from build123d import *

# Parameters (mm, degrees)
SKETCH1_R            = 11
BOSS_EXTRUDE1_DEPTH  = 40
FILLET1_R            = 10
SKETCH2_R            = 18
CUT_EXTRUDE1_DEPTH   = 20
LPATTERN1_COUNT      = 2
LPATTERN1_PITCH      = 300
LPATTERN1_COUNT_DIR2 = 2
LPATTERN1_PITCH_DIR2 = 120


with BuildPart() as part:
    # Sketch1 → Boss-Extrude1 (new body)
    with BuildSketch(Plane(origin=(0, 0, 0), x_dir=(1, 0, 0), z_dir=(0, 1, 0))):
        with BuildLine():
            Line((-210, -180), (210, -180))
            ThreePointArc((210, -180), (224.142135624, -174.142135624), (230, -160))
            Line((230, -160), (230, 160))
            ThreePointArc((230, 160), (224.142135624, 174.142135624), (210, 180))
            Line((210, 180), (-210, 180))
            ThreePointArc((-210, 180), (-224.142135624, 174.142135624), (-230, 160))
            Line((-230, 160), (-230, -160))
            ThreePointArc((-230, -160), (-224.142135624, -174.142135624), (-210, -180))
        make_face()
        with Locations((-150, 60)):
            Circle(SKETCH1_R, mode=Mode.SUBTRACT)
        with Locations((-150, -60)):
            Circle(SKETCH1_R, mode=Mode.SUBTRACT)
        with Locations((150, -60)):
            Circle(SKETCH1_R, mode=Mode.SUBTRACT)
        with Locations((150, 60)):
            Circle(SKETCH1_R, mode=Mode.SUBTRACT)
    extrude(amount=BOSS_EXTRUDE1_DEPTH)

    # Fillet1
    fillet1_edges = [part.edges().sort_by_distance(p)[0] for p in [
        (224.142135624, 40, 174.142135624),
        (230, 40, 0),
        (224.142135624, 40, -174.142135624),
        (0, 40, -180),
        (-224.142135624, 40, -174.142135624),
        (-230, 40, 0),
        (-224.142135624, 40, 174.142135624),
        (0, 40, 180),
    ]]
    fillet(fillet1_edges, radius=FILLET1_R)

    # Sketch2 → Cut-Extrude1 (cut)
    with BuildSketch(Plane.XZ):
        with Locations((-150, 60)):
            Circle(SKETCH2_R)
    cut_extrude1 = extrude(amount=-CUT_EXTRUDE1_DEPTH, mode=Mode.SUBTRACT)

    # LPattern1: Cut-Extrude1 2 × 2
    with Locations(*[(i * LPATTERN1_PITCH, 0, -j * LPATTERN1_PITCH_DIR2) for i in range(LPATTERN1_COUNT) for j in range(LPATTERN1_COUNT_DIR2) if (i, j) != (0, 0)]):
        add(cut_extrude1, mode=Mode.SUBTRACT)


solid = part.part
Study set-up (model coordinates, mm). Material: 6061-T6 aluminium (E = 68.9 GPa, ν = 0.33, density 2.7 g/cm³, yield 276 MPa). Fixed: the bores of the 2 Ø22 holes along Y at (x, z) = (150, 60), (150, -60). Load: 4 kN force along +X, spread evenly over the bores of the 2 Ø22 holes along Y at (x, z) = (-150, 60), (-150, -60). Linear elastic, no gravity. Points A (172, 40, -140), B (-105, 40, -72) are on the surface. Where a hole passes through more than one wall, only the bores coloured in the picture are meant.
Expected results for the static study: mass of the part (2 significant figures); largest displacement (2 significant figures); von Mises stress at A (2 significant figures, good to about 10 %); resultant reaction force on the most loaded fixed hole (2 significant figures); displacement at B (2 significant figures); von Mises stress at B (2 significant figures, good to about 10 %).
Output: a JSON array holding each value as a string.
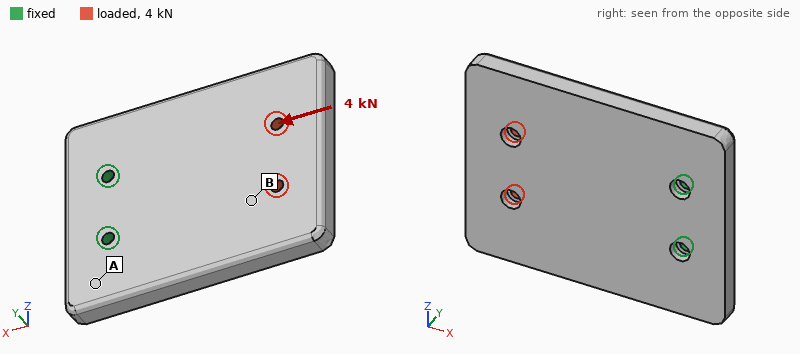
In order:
["17 kg", "19 µm", "0.20 MPa", "2.0 kN", "9.2 µm", "0.96 MPa"]
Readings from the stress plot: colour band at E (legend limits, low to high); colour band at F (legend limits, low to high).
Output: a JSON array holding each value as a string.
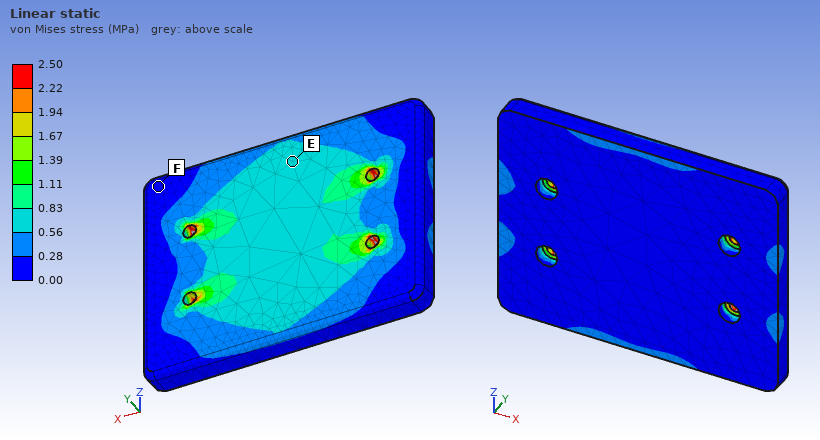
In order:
["0.56 to 0.83 MPa", "0.00 to 0.28 MPa"]
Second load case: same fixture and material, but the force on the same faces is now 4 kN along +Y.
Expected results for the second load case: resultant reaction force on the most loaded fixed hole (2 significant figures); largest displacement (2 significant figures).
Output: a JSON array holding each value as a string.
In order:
["2.5 kN", "0.76 mm"]
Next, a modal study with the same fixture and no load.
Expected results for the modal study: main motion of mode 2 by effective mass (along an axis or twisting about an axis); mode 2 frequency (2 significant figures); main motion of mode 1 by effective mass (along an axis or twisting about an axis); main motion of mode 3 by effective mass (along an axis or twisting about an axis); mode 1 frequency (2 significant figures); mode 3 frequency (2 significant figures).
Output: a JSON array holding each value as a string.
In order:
["twisting about X", "450 Hz", "along Y", "along Z", "160 Hz", "690 Hz"]
